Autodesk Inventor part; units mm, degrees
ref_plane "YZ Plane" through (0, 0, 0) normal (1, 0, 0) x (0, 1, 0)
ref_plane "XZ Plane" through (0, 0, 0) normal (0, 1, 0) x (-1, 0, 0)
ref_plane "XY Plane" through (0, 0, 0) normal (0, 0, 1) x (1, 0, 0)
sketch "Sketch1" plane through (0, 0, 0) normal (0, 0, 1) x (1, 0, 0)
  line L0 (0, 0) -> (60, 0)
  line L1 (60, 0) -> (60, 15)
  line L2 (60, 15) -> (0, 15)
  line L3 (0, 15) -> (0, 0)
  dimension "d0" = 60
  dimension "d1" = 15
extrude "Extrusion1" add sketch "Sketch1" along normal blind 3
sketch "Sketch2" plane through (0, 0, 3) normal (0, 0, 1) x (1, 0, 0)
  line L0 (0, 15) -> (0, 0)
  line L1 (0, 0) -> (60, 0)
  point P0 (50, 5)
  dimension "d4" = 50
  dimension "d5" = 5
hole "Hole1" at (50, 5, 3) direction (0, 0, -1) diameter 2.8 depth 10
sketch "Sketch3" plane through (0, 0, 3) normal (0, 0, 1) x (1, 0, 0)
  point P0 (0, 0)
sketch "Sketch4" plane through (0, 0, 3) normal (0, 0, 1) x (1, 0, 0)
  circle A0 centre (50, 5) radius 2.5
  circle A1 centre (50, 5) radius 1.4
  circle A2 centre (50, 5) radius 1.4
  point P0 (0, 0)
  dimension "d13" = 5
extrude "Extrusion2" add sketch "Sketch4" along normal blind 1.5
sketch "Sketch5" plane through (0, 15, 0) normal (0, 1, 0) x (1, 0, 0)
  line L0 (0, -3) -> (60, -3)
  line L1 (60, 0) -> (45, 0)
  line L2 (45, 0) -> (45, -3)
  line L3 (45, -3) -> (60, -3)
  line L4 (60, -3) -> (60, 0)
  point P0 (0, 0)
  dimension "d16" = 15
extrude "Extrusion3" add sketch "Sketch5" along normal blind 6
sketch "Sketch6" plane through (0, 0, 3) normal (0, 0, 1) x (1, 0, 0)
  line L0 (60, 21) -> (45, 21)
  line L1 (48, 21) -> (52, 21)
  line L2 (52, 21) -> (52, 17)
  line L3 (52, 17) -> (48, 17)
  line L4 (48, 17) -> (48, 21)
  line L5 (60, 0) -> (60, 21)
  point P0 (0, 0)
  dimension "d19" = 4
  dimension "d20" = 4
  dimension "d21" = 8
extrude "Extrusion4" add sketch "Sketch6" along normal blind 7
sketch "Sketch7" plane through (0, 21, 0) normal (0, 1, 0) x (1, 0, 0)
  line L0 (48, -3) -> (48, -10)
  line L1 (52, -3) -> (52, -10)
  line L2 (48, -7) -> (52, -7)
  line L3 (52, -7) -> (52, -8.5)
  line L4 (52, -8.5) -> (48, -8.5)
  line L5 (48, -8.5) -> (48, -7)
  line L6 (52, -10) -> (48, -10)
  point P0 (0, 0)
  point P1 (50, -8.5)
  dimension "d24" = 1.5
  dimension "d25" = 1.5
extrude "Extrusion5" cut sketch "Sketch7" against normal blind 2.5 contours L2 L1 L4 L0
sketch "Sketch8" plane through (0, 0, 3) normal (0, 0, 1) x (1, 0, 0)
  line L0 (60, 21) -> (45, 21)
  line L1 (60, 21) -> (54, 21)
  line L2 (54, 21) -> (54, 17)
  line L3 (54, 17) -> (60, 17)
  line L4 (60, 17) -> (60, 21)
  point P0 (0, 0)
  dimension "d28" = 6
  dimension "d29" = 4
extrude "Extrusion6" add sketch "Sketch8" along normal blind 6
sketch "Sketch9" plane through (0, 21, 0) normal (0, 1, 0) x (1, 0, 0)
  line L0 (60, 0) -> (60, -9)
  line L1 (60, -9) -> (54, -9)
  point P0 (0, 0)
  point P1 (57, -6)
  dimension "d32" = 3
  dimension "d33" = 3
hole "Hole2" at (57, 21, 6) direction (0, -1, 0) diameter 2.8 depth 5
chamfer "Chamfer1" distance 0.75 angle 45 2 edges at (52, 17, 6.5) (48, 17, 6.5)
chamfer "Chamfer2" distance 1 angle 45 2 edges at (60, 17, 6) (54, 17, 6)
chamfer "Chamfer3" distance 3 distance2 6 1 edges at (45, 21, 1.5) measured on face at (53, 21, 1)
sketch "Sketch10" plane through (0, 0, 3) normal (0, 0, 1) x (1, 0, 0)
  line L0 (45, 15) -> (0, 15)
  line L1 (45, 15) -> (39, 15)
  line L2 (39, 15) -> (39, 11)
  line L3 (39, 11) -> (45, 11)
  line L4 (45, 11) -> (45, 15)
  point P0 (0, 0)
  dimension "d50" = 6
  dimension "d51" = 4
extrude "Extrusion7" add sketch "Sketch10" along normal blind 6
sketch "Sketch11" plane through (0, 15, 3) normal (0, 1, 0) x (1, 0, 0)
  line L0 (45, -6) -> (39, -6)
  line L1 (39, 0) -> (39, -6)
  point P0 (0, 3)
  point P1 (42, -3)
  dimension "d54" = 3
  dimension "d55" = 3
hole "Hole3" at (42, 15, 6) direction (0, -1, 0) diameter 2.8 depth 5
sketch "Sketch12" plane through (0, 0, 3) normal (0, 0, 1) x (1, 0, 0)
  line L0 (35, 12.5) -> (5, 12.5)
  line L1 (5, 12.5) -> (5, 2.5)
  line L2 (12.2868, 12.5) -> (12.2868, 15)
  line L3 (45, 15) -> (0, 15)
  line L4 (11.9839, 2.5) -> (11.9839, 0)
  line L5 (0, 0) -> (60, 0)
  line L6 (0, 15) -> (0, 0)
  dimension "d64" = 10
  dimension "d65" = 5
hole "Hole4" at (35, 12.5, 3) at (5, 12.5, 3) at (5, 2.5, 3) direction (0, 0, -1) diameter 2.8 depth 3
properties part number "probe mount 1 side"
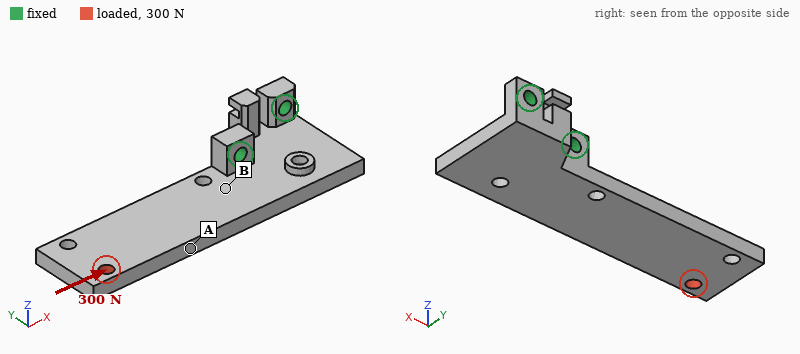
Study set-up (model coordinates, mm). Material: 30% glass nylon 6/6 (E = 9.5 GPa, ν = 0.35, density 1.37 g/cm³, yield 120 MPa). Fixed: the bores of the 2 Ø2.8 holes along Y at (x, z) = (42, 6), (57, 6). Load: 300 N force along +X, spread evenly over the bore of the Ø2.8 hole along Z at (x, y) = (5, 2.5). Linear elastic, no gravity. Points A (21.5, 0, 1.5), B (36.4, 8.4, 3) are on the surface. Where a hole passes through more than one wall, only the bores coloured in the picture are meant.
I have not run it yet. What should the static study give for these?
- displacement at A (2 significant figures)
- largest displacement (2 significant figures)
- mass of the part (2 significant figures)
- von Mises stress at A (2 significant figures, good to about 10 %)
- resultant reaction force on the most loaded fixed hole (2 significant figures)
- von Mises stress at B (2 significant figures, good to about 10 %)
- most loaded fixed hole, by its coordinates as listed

0.21 mm
0.44 mm
4.4 g
20 MPa
300 N
7.0 MPa
(42, 6)
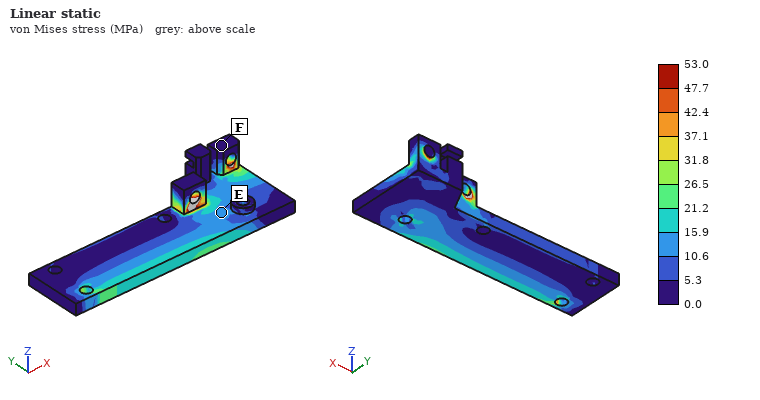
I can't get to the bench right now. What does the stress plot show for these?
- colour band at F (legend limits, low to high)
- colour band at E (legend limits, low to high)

0.0 to 5.3 MPa
10.6 to 15.9 MPa
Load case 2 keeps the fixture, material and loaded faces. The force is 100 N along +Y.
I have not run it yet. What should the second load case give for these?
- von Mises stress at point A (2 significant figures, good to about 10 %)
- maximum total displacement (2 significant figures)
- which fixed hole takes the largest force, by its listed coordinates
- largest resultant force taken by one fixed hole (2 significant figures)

15 MPa
0.65 mm
(42, 6)
300 N
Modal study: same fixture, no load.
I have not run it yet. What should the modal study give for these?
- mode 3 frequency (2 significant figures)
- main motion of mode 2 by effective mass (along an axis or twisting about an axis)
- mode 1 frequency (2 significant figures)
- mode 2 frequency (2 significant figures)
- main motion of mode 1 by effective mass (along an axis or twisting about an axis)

3000 Hz
along Y
670 Hz
2100 Hz
along Z
